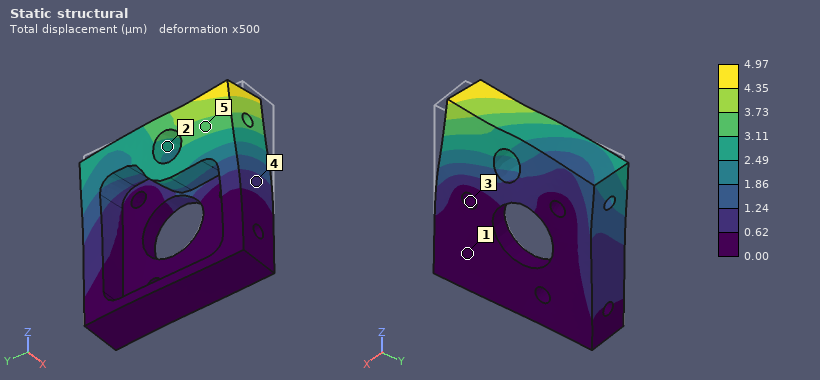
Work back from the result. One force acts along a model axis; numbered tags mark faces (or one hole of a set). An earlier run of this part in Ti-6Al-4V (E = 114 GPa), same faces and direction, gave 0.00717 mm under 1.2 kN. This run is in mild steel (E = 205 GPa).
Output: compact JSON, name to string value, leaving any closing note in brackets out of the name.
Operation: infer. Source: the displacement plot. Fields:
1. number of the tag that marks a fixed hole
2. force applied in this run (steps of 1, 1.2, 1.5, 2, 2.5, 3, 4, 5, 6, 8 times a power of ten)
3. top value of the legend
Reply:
{"number of the tag that marks a fixed hole": "3", "force applied in this run": "1.5 kN", "top value of the legend": "4.97 µm"}
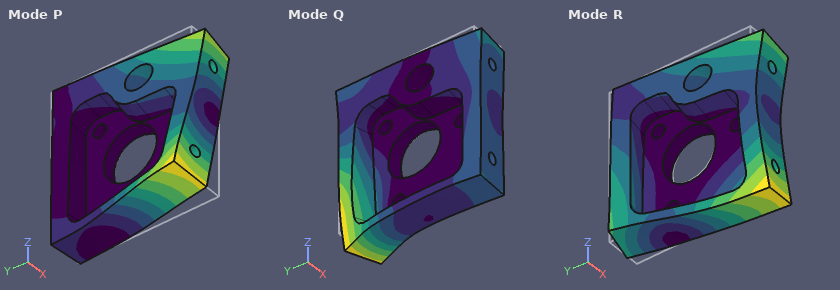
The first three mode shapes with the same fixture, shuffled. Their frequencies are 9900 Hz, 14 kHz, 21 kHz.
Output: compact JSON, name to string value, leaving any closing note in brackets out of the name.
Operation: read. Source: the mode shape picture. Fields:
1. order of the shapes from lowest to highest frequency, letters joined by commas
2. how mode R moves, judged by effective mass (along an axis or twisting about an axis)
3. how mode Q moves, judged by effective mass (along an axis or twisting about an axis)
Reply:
{"order of the shapes from lowest to highest frequency, letters joined by commas": "P, R, Q", "how mode R moves, judged by effective mass": "along X", "how mode Q moves, judged by effective mass": "along X"}
